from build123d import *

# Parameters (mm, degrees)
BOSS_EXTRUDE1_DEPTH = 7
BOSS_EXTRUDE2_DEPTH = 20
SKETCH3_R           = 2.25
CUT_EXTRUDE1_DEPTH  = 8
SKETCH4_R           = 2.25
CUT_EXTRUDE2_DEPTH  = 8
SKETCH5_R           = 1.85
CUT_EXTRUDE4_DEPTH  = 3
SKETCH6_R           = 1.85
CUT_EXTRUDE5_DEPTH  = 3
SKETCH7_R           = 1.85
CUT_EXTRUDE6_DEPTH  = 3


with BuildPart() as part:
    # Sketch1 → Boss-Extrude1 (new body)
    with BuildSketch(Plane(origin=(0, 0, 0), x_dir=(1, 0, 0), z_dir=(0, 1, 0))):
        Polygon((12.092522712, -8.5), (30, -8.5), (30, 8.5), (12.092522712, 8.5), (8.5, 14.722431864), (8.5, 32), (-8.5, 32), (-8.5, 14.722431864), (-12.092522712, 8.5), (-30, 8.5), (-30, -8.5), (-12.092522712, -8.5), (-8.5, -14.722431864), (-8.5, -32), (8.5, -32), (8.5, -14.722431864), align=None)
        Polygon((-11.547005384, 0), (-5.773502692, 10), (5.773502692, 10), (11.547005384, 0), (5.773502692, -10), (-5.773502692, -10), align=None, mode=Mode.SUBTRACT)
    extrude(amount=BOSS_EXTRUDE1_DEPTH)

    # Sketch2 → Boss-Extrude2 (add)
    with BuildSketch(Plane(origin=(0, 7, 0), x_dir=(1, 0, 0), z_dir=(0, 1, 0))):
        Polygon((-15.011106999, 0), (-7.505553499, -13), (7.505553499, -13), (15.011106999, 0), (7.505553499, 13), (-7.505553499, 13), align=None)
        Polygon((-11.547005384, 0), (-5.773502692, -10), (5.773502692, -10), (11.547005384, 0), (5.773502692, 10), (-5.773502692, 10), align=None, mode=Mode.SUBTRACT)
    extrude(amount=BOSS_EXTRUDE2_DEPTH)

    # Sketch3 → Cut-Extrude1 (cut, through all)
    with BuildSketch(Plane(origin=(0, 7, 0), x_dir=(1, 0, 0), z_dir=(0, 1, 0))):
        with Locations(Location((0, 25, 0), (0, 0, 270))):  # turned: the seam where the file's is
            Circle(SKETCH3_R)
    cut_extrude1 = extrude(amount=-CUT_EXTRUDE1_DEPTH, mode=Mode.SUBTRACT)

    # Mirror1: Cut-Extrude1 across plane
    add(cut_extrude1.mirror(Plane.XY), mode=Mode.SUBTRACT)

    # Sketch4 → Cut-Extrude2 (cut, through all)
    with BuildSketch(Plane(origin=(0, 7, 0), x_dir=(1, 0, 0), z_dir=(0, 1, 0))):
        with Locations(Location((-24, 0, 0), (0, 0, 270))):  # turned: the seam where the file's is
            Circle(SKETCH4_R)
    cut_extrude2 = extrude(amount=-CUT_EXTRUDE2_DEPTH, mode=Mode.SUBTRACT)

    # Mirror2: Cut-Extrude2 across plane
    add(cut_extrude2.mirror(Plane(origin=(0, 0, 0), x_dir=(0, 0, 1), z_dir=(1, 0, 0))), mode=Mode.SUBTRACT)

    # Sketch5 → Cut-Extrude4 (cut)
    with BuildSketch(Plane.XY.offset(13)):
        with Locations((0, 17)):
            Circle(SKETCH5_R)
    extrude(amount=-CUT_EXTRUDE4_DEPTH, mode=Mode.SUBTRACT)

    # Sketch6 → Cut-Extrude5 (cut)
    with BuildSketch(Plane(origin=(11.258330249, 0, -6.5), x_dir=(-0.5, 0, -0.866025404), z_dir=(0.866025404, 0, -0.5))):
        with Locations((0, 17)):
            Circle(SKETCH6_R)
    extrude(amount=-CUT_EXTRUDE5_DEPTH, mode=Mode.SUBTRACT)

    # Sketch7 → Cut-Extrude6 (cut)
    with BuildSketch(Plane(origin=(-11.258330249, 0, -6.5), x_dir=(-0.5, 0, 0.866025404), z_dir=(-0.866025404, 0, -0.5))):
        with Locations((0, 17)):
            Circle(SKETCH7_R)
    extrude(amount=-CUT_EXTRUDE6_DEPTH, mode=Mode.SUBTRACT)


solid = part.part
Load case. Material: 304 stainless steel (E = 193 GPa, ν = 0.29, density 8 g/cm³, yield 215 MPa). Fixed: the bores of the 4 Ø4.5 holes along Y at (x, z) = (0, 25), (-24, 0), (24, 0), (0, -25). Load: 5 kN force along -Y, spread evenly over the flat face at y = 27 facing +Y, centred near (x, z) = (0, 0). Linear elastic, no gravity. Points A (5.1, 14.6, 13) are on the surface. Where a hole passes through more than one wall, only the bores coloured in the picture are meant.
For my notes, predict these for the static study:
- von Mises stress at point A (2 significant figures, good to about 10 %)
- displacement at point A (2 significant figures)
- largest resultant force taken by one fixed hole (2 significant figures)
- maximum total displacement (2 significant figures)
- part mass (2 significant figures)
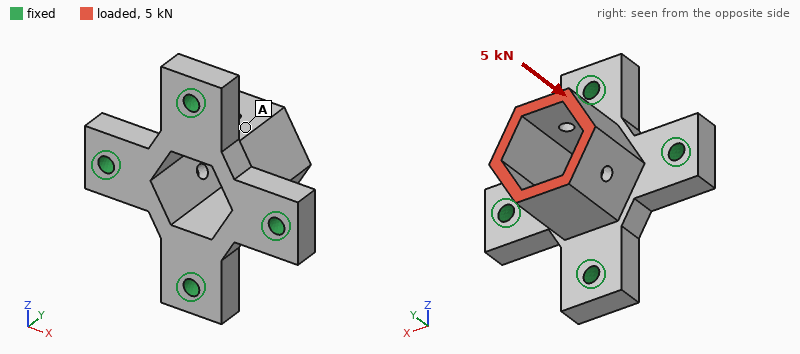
22 MPa
7.6 µm
1.4 kN
9.1 µm
120 g
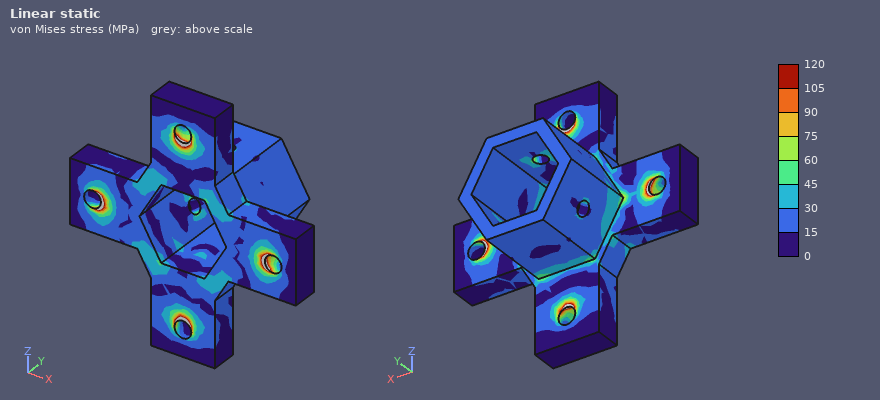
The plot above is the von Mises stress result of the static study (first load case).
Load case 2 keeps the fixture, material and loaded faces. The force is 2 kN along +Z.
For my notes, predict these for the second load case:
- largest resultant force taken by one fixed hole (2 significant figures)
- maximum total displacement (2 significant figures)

1.4 kN
20 µm
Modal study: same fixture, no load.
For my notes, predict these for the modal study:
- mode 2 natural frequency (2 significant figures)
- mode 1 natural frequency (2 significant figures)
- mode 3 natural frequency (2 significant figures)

14 kHz
14 kHz
16 kHz
